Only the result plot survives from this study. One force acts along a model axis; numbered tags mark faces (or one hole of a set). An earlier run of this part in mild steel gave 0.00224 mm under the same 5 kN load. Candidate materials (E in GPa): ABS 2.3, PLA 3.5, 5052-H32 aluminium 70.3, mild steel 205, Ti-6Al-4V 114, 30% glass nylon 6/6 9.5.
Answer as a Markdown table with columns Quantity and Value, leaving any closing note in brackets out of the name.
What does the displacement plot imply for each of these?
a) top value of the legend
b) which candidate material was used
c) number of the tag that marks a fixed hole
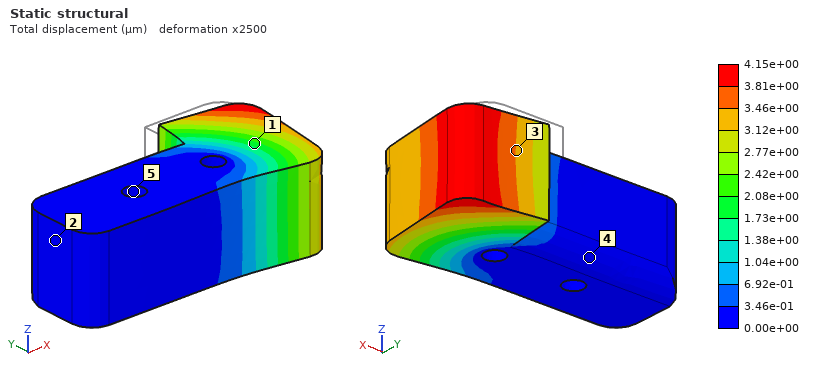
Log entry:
| Quantity | Value |
|---|---|
| top value of the legend | 4.15e+00 µm |
| which candidate material was used | Ti-6Al-4V |
| number of the tag that marks a fixed hole | 5 |
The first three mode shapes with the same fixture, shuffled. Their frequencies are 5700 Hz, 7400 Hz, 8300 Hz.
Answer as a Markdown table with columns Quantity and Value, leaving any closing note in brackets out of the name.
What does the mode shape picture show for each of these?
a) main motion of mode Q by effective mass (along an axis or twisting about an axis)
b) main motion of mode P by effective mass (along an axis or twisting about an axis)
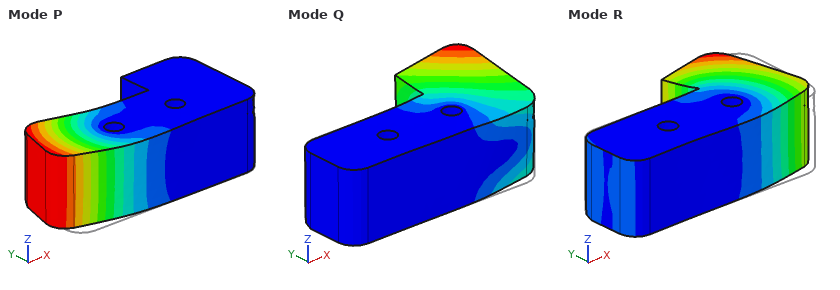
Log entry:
| Quantity | Value |
|---|---|
| main motion of mode Q by effective mass | along Z |
| main motion of mode P by effective mass | along Y |
